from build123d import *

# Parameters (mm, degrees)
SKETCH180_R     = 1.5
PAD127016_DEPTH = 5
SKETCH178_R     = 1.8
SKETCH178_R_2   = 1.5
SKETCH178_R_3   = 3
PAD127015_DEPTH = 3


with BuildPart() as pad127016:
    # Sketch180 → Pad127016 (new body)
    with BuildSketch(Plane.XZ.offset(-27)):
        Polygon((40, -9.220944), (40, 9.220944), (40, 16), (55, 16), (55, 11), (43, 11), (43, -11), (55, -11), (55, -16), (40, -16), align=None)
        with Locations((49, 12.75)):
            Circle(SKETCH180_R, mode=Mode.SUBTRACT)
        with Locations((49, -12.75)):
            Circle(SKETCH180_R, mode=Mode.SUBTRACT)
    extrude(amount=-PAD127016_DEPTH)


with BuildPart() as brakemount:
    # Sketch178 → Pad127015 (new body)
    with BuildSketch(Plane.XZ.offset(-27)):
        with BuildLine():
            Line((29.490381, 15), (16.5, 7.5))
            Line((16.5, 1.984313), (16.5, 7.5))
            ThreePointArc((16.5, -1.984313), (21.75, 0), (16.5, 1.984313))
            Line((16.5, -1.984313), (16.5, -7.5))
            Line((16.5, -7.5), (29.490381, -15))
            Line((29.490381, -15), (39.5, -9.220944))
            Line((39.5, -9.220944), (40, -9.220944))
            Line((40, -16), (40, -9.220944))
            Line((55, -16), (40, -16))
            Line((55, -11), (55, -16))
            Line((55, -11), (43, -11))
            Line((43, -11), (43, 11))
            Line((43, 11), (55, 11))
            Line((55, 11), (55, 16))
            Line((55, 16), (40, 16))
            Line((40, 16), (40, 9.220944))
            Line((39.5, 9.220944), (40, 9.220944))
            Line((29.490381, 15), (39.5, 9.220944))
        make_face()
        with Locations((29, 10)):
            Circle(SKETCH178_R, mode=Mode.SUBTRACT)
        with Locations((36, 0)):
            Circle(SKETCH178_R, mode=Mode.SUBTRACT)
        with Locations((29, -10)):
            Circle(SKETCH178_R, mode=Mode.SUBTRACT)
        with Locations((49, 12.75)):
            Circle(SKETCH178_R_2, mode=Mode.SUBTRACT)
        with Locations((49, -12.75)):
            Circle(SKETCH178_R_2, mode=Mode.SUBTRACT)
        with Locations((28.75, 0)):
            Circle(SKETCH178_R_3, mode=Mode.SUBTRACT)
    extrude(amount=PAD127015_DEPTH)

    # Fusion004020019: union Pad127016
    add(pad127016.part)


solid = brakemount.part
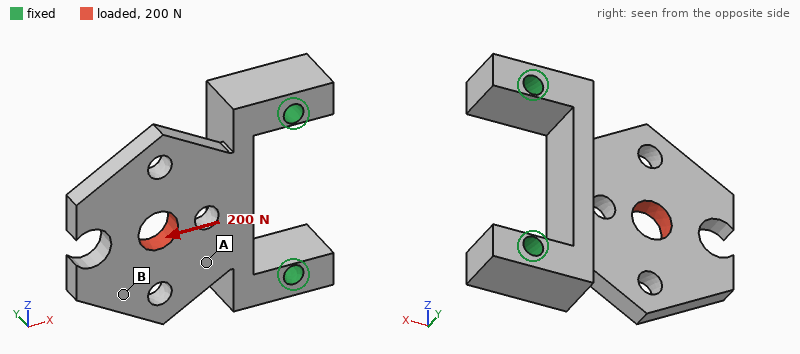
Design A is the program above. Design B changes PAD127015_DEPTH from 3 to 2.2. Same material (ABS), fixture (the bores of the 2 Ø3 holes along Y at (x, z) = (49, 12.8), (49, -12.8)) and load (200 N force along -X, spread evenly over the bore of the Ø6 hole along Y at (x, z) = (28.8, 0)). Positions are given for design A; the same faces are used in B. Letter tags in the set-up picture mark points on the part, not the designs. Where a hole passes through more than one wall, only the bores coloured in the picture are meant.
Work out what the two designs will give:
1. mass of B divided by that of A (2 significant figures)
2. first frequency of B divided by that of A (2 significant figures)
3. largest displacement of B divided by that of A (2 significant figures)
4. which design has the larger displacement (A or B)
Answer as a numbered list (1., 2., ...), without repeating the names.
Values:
1. 0.82
2. 0.86
3. 1.4
4. B
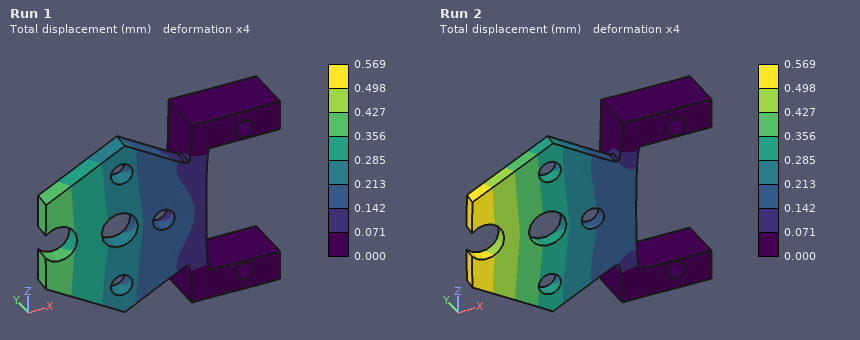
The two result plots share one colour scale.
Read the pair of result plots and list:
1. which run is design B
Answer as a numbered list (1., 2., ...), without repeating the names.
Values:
1. Run 2
